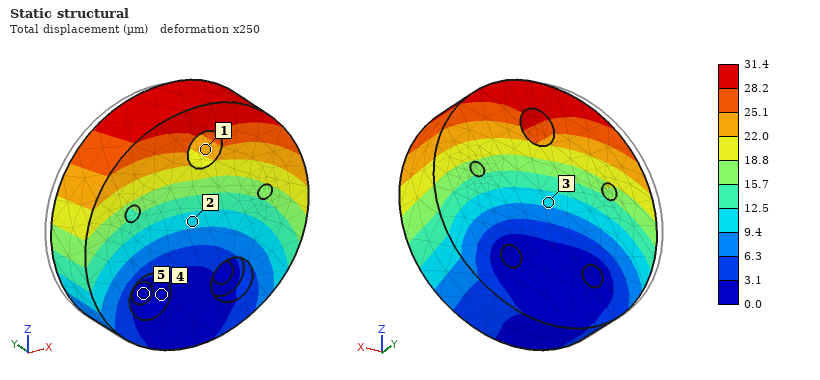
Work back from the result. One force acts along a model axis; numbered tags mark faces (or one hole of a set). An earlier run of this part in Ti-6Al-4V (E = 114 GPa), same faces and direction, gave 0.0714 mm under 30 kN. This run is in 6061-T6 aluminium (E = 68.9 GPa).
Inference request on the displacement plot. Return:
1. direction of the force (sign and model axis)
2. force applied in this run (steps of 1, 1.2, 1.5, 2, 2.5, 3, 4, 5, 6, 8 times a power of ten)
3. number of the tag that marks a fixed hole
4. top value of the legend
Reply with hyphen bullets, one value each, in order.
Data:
- +X
- 8 kN
- 5
- 31.4 µm
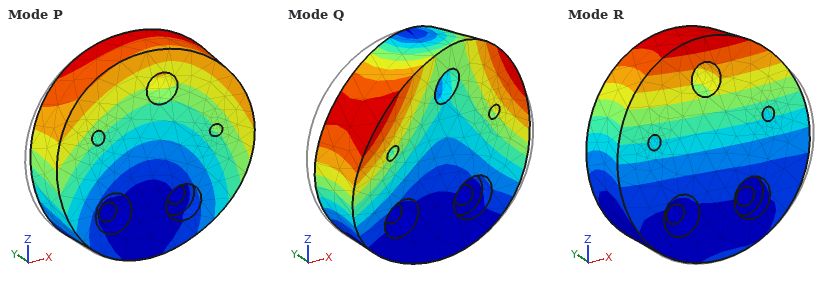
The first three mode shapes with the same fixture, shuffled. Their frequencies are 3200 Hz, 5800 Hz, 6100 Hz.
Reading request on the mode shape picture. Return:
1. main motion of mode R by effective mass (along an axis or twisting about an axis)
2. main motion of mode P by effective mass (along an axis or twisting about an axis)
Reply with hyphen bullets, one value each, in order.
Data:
- along Y
- along X
